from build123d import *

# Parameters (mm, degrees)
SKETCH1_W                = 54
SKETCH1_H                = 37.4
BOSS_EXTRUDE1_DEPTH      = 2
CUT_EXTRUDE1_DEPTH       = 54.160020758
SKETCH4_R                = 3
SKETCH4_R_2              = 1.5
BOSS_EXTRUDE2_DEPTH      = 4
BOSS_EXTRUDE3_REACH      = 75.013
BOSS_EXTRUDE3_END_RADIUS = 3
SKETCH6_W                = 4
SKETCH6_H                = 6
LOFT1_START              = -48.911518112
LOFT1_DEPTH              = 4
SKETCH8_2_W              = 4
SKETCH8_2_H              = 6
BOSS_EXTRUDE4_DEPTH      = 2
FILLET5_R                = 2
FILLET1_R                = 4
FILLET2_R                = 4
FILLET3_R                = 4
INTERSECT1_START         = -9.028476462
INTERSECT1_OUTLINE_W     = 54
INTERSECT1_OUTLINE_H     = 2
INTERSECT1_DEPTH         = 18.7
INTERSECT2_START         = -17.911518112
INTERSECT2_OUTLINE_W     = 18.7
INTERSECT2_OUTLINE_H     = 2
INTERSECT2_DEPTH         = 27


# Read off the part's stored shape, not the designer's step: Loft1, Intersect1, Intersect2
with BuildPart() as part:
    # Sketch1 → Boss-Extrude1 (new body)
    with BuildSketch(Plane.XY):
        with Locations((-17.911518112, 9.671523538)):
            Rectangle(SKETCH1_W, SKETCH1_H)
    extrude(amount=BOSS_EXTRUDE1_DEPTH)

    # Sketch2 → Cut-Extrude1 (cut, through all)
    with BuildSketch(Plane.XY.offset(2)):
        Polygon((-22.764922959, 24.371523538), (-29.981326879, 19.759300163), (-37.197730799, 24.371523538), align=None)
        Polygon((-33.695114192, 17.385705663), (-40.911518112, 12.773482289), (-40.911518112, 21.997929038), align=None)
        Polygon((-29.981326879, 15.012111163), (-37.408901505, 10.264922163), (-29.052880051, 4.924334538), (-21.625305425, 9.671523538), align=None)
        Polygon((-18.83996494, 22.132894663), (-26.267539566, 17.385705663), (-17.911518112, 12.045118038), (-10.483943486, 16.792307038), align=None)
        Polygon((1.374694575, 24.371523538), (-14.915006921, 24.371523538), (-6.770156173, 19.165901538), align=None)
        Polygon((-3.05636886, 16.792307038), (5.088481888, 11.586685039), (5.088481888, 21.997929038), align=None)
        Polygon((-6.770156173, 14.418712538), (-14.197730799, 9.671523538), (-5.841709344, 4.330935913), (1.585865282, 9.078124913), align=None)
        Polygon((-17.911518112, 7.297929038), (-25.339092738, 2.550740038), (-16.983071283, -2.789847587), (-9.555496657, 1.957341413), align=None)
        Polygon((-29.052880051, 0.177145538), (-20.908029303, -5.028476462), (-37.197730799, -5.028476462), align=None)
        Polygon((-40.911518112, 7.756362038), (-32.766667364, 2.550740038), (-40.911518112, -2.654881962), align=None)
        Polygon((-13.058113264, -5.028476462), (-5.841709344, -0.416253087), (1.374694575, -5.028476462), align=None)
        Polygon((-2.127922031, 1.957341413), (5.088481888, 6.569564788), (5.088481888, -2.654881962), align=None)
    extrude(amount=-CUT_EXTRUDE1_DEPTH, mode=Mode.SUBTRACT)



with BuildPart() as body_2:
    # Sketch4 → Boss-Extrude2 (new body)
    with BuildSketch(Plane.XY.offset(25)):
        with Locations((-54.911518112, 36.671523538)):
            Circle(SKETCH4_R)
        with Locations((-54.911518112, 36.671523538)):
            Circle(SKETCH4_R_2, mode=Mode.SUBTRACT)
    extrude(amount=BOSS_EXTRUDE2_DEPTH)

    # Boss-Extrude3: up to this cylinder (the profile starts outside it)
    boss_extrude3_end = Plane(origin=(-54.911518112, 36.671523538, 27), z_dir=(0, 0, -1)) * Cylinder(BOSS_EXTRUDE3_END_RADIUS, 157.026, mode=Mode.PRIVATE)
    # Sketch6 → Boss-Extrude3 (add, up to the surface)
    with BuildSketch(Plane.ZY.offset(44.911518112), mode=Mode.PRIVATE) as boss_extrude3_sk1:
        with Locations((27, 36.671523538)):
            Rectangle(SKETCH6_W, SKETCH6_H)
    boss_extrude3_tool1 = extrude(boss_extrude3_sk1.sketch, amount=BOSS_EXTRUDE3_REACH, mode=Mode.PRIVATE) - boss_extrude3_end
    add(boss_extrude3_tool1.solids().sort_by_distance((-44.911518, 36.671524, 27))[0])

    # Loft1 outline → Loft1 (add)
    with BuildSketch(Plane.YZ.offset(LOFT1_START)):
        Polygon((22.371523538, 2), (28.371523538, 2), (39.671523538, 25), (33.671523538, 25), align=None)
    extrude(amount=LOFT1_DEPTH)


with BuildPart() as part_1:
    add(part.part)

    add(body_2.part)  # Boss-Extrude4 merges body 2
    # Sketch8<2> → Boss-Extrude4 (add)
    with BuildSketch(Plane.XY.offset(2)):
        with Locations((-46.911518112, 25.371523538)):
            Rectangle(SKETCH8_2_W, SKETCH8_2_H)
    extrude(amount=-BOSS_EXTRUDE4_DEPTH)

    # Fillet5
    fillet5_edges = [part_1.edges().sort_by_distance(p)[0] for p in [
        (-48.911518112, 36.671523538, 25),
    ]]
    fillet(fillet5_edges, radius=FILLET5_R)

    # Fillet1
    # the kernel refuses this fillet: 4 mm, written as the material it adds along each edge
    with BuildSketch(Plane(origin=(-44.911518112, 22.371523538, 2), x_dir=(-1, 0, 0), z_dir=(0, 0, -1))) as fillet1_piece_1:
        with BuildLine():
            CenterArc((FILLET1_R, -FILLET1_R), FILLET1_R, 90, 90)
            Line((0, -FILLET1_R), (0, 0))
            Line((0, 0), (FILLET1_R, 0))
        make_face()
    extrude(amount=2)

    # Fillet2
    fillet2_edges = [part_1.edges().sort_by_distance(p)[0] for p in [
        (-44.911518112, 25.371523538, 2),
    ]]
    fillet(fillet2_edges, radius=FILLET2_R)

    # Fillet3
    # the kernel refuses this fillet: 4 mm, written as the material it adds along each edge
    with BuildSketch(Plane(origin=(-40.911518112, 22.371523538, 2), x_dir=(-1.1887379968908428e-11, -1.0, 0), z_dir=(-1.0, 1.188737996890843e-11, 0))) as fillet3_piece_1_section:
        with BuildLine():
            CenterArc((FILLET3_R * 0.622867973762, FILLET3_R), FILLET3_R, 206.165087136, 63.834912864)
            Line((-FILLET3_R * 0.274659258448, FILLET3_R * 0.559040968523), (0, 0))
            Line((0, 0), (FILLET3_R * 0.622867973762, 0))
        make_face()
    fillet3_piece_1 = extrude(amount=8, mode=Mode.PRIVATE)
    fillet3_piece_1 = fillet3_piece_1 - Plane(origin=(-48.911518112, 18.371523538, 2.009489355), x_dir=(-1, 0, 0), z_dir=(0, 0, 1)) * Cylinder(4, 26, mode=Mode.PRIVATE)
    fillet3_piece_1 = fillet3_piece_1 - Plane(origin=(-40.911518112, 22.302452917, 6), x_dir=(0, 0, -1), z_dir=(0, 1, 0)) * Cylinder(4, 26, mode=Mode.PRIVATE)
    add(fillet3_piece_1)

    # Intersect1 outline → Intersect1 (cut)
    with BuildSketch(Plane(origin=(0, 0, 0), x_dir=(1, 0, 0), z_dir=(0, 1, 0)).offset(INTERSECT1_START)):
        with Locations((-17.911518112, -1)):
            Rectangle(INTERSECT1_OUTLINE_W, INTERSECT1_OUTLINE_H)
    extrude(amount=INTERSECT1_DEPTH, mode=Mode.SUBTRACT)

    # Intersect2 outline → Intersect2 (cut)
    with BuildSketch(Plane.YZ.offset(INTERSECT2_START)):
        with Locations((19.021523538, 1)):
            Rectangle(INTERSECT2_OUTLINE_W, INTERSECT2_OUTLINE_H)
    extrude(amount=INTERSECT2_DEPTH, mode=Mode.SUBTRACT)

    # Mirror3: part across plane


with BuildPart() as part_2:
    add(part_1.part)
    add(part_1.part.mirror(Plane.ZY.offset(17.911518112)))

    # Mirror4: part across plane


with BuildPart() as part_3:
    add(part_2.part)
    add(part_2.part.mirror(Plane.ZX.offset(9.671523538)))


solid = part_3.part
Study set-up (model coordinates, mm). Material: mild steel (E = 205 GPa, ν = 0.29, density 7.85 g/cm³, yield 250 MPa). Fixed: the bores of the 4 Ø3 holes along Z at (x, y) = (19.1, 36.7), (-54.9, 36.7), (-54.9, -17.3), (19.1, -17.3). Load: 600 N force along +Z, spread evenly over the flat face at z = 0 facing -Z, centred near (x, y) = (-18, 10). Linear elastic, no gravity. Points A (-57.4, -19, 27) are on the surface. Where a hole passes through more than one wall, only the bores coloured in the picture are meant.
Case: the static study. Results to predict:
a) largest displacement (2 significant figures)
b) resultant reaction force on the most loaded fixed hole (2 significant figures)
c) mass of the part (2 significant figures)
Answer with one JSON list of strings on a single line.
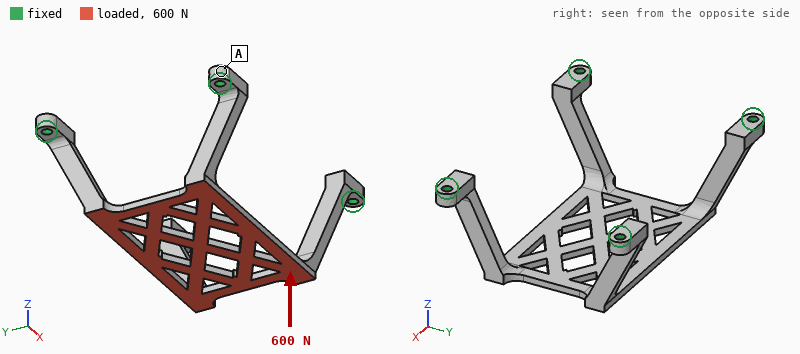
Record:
["0.11 mm", "190 N", "50 g"]
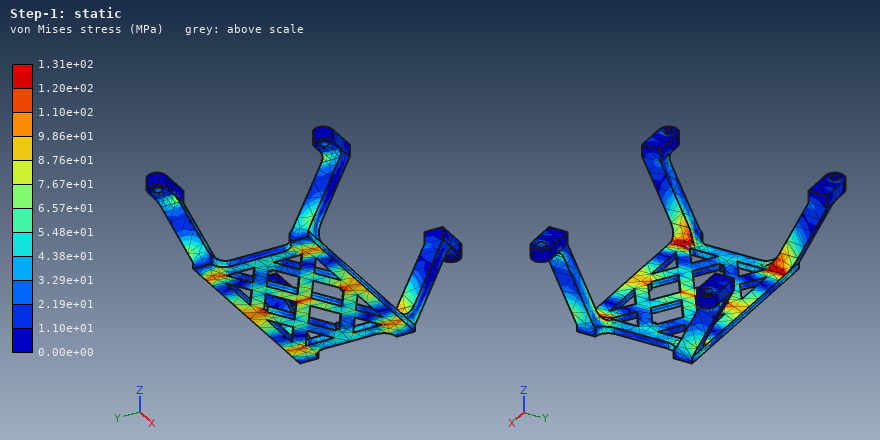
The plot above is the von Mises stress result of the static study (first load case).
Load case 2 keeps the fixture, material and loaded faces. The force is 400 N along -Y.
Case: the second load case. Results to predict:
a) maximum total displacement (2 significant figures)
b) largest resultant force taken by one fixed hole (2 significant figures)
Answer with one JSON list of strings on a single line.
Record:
["51 µm", "120 N"]
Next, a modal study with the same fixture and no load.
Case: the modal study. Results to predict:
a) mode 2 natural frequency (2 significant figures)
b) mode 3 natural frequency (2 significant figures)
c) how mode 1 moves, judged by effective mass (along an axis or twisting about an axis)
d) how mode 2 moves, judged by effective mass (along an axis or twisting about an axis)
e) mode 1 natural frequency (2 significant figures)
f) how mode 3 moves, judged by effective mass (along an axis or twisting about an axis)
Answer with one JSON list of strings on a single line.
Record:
["2500 Hz", "2900 Hz", "along X", "along Y", "1900 Hz", "along Z"]
